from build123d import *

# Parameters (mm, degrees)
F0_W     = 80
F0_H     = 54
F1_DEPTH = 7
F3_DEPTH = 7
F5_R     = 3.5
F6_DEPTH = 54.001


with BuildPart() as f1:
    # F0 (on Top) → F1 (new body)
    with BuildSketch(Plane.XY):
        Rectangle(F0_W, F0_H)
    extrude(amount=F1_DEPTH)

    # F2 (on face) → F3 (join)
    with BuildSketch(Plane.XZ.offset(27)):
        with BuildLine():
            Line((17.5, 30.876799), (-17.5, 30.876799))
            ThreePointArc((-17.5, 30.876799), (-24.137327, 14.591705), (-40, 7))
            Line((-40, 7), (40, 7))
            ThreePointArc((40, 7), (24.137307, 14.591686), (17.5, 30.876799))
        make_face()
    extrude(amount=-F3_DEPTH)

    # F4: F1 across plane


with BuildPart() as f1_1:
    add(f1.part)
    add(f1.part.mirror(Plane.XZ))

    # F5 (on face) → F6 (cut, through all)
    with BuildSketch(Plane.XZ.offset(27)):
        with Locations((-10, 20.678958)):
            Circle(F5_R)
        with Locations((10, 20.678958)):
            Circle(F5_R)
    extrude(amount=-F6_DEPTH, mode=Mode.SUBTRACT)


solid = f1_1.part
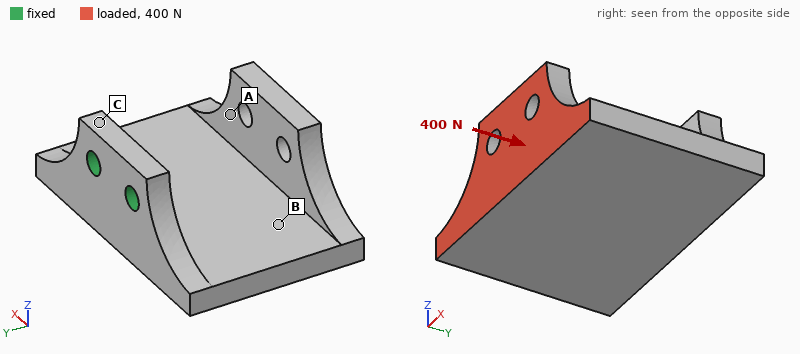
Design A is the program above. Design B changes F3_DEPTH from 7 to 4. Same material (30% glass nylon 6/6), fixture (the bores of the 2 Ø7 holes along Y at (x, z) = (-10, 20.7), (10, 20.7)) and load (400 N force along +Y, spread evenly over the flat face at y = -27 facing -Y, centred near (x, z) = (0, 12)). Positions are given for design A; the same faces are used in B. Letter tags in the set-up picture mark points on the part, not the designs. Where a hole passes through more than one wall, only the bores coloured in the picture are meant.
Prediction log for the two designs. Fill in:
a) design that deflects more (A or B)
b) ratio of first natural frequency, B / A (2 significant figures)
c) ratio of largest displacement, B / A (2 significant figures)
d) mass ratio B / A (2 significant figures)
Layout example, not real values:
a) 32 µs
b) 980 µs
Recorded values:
a) B
b) 0.55
c) 1.6
d) 0.86
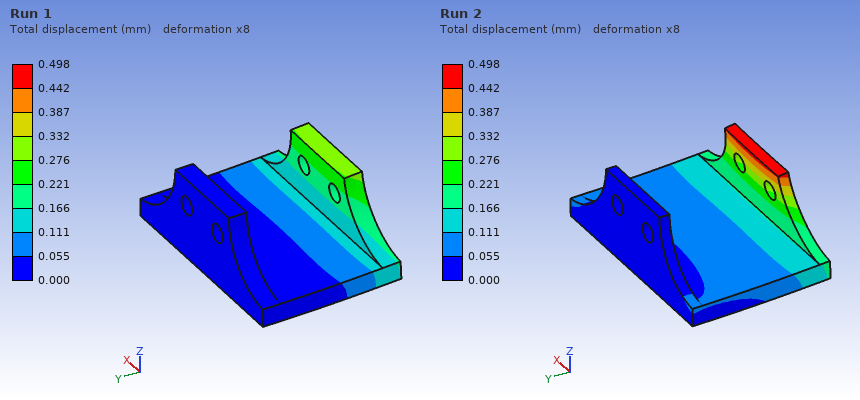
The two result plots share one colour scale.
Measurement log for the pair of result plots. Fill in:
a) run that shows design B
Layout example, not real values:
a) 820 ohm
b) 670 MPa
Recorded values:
a) Run 2
